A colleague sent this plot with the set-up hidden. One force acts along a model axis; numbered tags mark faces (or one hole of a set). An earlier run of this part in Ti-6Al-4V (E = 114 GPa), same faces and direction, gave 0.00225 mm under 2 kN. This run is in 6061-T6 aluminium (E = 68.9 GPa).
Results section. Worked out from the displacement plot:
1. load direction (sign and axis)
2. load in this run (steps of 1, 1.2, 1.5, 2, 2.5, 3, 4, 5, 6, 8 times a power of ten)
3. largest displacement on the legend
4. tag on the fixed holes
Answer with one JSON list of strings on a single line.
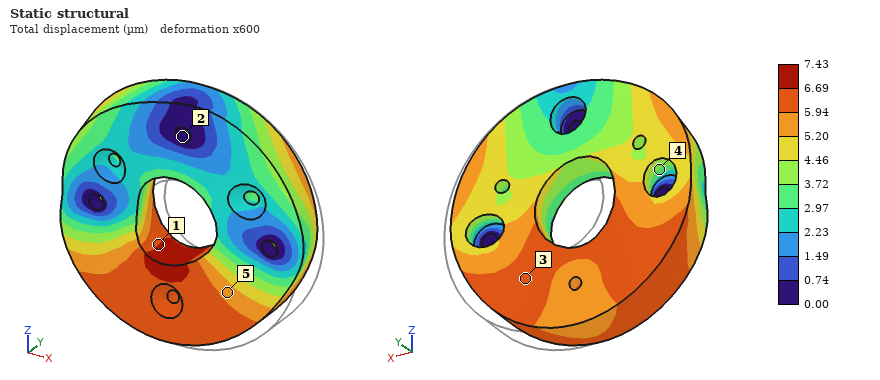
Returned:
["-X", "4 kN", "7.43 µm", "2"]
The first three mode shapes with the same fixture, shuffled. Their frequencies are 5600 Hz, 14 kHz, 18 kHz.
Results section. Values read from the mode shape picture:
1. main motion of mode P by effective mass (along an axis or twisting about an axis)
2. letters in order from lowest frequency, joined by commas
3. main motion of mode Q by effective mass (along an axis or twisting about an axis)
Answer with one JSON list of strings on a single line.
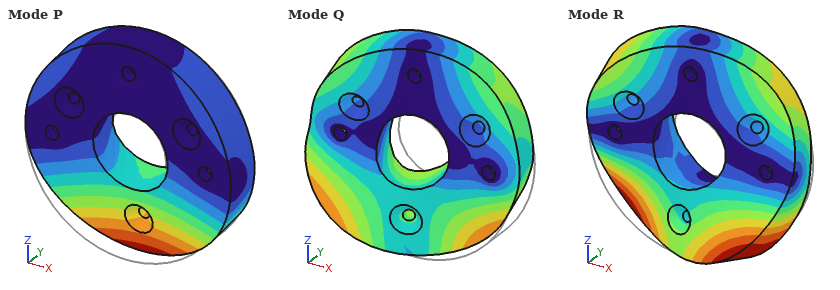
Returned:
["along Y", "P, R, Q", "along X"]
